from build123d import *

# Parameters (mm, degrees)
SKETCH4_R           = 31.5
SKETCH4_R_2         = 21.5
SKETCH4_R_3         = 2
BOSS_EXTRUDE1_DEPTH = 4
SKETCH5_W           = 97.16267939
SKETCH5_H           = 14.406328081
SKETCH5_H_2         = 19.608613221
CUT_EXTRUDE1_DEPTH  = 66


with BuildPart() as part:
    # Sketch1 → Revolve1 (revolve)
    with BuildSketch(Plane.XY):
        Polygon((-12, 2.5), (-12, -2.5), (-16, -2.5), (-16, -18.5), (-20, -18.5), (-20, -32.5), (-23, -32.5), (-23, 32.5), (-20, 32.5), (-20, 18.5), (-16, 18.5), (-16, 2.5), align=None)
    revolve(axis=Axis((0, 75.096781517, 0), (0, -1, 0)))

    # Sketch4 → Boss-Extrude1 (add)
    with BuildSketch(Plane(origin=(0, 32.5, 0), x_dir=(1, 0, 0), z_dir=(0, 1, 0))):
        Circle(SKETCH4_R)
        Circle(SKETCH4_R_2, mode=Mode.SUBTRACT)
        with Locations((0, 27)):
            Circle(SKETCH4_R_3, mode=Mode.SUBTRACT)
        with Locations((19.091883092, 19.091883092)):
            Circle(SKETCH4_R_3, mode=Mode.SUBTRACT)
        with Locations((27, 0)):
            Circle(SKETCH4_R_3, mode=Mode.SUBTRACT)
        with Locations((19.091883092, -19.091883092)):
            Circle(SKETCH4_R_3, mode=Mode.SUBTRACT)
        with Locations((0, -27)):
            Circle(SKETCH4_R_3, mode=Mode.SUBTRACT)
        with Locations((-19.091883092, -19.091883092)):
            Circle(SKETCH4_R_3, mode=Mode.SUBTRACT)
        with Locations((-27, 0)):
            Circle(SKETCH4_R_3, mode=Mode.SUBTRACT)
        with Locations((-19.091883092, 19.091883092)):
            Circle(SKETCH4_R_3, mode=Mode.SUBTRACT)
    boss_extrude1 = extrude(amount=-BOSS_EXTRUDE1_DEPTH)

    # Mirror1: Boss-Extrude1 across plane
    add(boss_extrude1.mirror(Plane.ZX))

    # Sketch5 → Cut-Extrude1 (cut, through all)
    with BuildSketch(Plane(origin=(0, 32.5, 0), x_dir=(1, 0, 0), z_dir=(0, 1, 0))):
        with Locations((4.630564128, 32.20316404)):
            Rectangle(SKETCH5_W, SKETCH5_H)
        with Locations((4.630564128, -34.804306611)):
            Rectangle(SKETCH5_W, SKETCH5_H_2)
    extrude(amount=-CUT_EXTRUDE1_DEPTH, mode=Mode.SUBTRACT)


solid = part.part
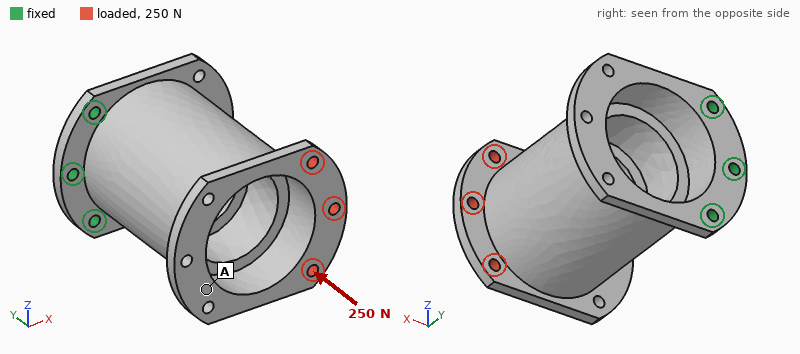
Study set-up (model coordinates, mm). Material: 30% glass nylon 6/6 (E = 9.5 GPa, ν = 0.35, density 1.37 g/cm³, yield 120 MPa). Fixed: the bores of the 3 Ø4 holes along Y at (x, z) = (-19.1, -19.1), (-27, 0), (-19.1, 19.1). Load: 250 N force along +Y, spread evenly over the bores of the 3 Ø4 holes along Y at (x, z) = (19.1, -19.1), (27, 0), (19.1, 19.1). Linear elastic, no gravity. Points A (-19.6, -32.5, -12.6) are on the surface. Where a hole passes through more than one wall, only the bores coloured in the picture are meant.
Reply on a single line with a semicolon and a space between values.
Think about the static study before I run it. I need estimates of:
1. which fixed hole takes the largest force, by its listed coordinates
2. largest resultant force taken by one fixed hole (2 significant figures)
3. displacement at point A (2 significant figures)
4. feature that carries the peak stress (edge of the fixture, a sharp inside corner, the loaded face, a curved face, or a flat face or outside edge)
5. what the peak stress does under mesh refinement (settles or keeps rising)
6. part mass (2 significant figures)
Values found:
(-27, 0); 700 N; 0.84 mm; edge of the fixture; keeps rising; 73 g
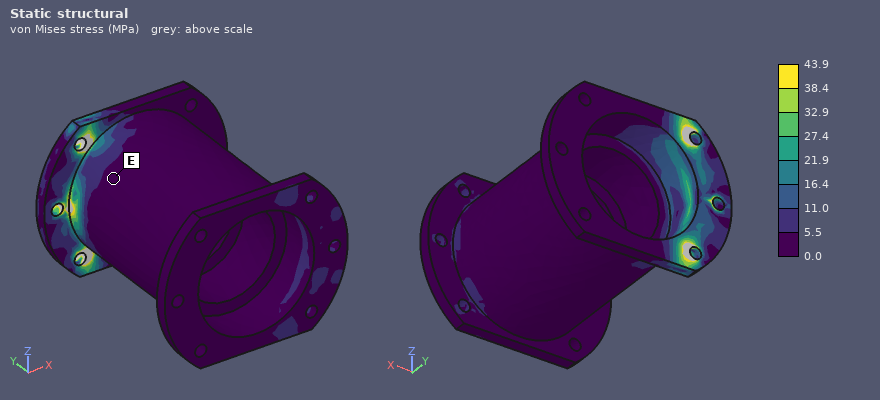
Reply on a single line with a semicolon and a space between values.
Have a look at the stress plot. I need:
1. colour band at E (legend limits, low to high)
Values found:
0.0 to 5.5 MPa
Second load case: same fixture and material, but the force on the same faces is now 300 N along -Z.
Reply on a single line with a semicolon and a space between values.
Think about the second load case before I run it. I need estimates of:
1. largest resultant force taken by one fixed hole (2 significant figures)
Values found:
610 N
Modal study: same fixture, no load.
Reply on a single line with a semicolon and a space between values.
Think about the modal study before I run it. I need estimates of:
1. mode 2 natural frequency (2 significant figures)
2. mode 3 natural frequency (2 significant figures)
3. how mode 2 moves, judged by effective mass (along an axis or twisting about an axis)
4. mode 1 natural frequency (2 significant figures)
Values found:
1100 Hz; 1600 Hz; along Z; 370 Hz
